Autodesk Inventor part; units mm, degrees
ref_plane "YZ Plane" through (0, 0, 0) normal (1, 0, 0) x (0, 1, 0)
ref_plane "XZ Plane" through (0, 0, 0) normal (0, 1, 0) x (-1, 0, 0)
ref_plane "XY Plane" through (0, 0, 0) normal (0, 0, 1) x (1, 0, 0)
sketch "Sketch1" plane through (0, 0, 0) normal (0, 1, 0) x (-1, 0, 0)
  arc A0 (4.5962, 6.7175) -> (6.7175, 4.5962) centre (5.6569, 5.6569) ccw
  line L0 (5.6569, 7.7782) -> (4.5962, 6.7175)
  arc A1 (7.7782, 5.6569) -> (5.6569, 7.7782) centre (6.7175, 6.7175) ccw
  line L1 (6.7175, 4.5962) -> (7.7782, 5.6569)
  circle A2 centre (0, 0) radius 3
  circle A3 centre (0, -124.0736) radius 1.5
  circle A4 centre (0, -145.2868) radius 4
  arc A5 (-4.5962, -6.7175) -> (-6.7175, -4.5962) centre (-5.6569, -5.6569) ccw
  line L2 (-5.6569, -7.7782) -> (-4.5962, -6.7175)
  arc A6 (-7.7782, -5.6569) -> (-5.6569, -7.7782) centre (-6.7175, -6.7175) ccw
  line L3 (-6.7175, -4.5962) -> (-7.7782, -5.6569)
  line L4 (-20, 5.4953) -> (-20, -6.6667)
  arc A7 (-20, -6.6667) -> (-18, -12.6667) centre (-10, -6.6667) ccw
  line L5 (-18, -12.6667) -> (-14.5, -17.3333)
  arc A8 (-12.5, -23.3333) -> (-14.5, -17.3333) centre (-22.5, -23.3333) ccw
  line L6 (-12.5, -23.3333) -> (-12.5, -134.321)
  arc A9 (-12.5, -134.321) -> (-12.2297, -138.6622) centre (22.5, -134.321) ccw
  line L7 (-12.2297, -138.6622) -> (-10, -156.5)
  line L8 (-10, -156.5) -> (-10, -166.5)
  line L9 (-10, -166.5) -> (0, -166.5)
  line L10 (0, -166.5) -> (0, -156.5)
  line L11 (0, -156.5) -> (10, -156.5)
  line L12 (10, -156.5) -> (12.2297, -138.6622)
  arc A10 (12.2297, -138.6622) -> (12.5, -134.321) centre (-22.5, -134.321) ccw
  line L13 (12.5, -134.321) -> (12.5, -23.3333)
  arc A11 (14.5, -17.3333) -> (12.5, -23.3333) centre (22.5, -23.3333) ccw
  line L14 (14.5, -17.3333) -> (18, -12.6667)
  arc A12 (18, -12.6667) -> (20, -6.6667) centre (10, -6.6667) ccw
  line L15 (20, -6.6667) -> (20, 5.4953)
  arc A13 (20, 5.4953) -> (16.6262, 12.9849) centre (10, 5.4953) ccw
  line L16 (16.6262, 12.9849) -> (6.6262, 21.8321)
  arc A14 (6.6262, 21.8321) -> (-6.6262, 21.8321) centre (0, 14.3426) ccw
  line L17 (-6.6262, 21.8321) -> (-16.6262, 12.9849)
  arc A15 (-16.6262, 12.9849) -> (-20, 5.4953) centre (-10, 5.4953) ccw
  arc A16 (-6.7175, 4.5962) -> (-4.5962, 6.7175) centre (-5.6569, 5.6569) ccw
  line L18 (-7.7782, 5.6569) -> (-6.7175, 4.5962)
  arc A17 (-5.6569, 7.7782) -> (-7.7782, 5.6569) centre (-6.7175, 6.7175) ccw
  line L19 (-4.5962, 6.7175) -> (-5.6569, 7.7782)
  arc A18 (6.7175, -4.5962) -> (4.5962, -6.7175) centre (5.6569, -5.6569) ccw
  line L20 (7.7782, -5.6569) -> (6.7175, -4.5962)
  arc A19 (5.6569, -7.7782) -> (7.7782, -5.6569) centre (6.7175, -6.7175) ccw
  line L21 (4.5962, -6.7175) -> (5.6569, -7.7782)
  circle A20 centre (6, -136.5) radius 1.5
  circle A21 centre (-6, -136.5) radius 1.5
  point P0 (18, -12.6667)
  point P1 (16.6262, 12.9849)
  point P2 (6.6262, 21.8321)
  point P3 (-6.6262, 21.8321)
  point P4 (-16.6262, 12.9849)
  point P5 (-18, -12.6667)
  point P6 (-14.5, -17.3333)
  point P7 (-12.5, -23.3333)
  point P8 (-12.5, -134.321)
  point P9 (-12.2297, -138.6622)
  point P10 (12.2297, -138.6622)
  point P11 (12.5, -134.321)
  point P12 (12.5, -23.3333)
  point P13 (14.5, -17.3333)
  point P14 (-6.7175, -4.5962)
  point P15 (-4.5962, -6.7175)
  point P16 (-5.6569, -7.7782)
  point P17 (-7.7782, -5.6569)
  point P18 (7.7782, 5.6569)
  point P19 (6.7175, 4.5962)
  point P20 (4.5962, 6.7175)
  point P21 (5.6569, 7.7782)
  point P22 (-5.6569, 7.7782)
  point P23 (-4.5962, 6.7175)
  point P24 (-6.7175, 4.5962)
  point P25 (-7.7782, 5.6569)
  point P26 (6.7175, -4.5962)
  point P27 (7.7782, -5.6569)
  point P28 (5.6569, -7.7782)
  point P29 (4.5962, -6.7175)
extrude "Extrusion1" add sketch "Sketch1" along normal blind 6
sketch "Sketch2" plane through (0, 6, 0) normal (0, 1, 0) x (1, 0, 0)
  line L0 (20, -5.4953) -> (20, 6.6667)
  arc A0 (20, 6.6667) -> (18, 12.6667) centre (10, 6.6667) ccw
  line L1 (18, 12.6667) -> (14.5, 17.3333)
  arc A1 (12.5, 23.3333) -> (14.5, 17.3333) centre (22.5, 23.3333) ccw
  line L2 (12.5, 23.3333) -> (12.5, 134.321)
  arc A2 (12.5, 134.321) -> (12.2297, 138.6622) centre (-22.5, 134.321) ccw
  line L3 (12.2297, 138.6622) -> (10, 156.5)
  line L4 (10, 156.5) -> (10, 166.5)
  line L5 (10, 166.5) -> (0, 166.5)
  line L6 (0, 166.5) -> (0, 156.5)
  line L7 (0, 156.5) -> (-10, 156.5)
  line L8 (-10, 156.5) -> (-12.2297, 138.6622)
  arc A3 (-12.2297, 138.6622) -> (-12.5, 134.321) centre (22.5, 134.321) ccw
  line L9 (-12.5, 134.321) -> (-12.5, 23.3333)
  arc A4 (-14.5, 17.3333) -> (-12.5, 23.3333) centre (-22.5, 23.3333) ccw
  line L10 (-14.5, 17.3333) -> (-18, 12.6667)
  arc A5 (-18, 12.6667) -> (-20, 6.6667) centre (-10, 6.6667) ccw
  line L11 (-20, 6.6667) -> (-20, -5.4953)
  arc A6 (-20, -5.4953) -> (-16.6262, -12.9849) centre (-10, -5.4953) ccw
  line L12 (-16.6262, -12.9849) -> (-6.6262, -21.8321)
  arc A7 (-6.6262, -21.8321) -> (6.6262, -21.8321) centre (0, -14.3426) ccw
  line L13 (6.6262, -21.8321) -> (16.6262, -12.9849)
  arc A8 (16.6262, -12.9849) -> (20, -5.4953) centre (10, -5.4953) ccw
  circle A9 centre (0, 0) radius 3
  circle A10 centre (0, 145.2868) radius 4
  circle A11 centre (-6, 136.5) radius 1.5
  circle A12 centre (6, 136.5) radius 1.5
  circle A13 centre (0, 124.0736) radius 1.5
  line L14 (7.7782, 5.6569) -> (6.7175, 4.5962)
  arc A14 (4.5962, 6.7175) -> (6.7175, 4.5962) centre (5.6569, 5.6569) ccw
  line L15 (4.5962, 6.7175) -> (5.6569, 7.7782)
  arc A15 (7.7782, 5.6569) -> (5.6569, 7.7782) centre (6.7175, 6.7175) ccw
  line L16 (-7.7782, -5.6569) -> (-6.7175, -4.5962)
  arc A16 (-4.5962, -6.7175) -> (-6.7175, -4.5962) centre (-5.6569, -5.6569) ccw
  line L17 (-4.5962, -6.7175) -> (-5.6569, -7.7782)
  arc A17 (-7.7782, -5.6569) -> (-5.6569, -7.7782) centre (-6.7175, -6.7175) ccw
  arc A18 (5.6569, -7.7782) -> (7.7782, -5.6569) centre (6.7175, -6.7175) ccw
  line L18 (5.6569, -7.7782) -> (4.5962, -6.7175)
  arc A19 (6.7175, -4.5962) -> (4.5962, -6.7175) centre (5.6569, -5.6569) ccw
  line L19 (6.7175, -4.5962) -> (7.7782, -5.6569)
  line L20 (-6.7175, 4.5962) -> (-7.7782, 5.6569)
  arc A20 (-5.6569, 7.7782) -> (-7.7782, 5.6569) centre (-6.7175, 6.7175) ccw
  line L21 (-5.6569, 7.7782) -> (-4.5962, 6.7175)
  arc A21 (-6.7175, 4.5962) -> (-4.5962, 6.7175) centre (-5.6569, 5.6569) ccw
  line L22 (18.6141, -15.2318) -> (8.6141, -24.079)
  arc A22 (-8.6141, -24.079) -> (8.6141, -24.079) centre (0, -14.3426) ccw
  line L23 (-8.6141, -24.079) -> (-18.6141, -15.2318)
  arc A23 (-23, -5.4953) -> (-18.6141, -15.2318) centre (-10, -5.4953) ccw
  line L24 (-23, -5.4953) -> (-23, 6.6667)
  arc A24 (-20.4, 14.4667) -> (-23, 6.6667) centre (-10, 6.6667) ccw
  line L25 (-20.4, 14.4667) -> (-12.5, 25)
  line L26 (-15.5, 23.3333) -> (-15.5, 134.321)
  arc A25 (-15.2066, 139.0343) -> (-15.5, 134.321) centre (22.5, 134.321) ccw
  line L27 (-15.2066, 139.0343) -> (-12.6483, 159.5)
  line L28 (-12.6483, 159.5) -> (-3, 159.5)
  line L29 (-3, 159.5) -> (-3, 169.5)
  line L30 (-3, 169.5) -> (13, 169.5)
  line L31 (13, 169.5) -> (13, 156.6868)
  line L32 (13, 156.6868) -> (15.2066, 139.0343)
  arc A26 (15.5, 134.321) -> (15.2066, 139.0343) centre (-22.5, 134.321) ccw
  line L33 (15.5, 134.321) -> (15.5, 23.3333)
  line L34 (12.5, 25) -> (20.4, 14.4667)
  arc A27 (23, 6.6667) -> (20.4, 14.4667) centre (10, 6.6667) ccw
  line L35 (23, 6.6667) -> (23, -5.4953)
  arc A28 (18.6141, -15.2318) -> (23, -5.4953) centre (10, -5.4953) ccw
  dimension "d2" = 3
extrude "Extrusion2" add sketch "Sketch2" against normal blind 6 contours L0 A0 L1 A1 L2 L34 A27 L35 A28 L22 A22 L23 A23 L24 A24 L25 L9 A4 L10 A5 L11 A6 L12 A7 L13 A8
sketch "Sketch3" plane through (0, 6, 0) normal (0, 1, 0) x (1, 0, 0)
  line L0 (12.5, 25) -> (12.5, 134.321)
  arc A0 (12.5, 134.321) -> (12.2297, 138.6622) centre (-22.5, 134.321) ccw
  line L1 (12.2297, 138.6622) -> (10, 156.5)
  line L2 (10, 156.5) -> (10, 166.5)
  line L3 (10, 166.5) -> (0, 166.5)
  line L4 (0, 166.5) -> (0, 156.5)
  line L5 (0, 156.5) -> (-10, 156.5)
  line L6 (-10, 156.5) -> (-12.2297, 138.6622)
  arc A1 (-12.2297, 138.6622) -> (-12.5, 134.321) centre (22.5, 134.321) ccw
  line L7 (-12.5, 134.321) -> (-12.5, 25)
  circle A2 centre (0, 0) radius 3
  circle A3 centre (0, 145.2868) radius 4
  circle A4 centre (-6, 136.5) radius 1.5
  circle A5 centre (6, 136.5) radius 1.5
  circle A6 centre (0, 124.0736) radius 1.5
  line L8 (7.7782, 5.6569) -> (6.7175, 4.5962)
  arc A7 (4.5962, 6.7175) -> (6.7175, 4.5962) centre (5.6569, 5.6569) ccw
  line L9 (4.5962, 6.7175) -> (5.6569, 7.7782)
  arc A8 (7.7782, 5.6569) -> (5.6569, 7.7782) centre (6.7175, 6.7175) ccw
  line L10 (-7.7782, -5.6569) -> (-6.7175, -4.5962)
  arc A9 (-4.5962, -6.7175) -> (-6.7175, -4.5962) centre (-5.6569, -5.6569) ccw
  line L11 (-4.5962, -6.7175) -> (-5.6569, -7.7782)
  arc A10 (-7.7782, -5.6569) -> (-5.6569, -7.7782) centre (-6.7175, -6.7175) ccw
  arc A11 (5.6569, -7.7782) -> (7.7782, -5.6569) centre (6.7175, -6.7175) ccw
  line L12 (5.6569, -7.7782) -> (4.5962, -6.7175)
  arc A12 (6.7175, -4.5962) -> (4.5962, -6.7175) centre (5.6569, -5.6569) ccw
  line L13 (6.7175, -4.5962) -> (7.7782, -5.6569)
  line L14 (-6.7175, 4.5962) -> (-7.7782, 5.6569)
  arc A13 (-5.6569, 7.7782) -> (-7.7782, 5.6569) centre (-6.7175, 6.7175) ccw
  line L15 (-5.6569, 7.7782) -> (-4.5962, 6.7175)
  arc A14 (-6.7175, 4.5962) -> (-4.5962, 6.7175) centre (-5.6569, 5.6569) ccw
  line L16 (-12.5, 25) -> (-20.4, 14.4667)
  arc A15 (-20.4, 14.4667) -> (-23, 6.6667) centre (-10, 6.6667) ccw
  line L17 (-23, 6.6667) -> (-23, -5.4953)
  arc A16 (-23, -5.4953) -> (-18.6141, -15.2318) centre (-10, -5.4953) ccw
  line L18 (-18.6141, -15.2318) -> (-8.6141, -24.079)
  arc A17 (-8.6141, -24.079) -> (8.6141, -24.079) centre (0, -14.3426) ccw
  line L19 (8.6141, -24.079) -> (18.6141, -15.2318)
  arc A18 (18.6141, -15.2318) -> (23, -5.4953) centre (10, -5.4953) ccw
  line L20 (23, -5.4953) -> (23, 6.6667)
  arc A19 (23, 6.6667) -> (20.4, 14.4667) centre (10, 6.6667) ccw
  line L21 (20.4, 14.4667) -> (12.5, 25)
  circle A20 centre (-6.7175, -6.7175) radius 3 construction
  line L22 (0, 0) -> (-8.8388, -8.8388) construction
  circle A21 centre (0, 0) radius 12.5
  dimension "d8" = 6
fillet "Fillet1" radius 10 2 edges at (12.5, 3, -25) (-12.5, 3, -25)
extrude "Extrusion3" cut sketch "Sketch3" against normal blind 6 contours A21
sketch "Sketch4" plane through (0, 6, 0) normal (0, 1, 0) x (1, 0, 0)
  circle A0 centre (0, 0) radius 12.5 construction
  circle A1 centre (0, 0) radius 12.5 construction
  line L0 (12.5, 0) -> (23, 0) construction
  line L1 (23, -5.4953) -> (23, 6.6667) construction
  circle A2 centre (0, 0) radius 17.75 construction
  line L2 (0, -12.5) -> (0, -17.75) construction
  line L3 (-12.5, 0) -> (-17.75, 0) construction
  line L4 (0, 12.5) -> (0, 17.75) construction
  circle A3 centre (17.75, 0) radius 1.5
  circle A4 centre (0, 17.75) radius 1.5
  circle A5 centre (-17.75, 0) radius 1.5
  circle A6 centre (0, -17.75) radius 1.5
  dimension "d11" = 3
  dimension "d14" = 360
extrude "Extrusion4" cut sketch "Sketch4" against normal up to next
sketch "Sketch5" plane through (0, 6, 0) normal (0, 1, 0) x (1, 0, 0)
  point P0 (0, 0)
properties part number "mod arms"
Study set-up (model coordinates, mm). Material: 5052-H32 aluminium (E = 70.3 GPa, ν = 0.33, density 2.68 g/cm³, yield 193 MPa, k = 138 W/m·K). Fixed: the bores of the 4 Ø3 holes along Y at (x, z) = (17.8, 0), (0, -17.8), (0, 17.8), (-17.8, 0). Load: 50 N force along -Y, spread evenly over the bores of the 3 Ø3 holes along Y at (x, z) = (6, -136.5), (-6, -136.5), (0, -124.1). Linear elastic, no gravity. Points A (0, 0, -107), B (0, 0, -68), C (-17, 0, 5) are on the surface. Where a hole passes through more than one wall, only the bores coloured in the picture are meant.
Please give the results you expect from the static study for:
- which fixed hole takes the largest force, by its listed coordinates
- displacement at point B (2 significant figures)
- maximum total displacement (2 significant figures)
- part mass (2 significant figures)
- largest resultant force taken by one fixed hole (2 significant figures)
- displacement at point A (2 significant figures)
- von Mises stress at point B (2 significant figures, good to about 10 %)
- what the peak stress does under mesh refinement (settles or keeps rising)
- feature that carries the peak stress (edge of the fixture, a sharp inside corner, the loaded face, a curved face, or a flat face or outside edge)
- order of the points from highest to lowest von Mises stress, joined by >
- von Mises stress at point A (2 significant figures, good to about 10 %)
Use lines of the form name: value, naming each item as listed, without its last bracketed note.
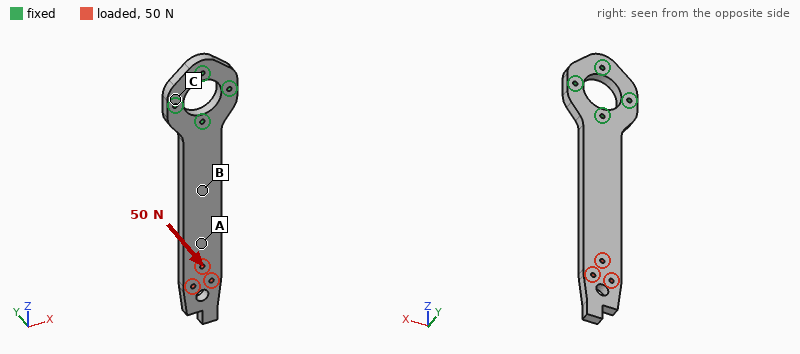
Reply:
which fixed hole takes the largest force, by its listed coordinates: (0, -17.8)
displacement at point B: 0.20 mm
maximum total displacement: 1.2 mm
part mass: 76 g
largest resultant force taken by one fixed hole: 200 N
displacement at point A: 0.54 mm
von Mises stress at point B: 21 MPa
what the peak stress does under mesh refinement: keeps rising
feature that carries the peak stress: edge of the fixture
order of the points from highest to lowest von Mises stress, joined by >: B > A > C
von Mises stress at point A: 8.5 MPa
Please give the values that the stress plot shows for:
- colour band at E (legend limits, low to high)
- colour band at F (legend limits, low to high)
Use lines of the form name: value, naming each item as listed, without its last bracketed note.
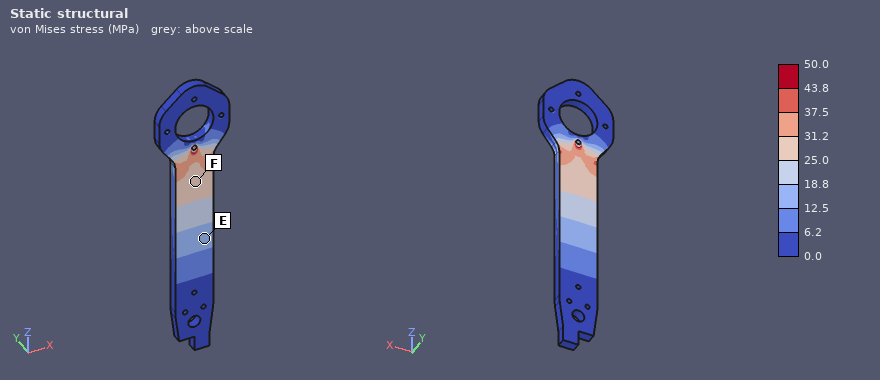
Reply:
colour band at E: 12.5 to 18.8 MPa
colour band at F: 25.0 to 31.2 MPa
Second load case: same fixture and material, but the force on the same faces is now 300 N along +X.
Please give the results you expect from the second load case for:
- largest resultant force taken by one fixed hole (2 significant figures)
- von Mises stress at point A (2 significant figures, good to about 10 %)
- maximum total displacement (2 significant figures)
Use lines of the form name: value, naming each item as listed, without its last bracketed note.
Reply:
largest resultant force taken by one fixed hole: 1.1 kN
von Mises stress at point A: 5.3 MPa
maximum total displacement: 0.45 mm
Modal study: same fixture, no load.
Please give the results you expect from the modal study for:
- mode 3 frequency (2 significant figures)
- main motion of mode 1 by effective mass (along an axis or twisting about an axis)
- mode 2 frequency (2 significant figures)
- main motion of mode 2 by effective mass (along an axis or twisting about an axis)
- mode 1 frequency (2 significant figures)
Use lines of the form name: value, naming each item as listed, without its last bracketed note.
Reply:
mode 3 frequency: 1500 Hz
main motion of mode 1 by effective mass: along Y
mode 2 frequency: 980 Hz
main motion of mode 2 by effective mass: along X
mode 1 frequency: 250 Hz
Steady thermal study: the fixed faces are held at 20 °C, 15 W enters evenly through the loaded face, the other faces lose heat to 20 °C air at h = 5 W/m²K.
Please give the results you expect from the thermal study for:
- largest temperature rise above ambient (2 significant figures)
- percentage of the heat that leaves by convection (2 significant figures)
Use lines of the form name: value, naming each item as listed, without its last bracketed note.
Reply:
largest temperature rise above ambient: 77 K
percentage of the heat that leaves by convection: 14 %
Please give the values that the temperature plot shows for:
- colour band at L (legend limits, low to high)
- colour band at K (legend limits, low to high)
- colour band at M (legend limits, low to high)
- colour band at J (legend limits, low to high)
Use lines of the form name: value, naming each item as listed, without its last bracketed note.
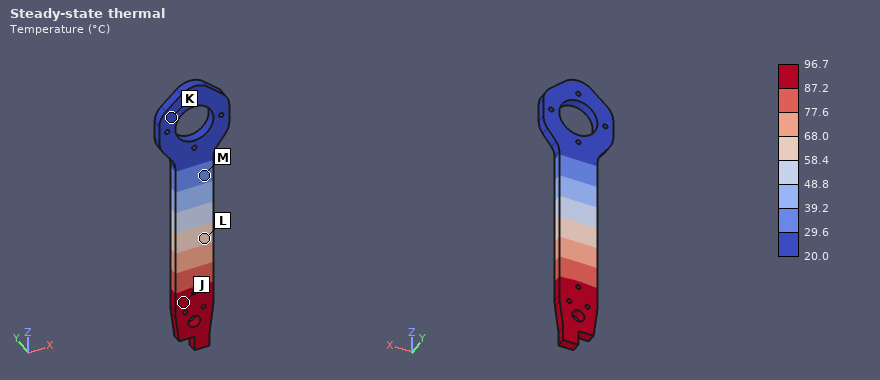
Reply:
colour band at L: 58.4 to 68.0 °C
colour band at K: 20.0 to 29.6 °C
colour band at M: 29.6 to 39.2 °C
colour band at J: 87.2 to 96.7 °C
